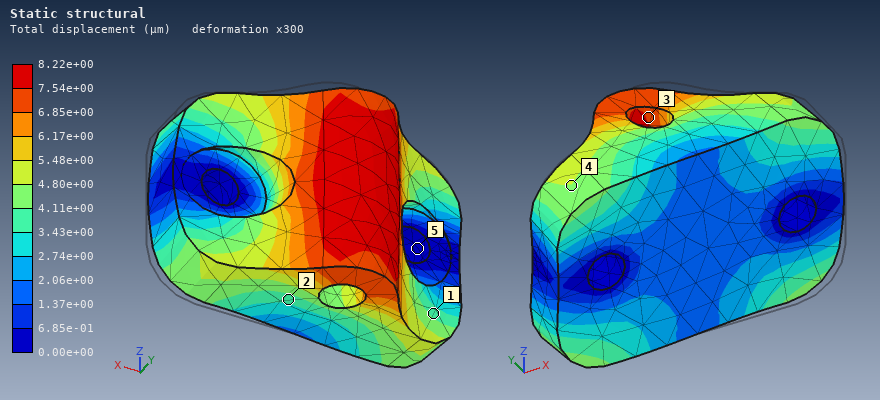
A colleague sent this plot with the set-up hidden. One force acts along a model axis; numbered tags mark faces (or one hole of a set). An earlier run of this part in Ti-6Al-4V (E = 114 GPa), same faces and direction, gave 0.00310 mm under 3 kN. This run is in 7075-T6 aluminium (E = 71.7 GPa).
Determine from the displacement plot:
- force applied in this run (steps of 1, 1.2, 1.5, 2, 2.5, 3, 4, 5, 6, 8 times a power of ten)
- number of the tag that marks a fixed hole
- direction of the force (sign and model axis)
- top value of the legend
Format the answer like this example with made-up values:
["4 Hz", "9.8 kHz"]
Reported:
["5 kN", "5", "-X", "8.22e+00 µm"]
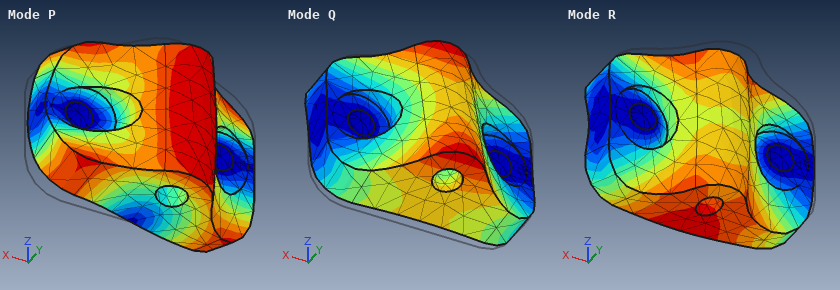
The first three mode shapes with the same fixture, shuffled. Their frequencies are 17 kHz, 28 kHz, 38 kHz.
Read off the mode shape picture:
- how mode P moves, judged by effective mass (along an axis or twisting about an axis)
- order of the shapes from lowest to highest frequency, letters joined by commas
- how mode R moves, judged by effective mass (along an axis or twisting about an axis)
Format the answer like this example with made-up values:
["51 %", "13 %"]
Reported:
["along X", "Q, R, P", "along Y"]
